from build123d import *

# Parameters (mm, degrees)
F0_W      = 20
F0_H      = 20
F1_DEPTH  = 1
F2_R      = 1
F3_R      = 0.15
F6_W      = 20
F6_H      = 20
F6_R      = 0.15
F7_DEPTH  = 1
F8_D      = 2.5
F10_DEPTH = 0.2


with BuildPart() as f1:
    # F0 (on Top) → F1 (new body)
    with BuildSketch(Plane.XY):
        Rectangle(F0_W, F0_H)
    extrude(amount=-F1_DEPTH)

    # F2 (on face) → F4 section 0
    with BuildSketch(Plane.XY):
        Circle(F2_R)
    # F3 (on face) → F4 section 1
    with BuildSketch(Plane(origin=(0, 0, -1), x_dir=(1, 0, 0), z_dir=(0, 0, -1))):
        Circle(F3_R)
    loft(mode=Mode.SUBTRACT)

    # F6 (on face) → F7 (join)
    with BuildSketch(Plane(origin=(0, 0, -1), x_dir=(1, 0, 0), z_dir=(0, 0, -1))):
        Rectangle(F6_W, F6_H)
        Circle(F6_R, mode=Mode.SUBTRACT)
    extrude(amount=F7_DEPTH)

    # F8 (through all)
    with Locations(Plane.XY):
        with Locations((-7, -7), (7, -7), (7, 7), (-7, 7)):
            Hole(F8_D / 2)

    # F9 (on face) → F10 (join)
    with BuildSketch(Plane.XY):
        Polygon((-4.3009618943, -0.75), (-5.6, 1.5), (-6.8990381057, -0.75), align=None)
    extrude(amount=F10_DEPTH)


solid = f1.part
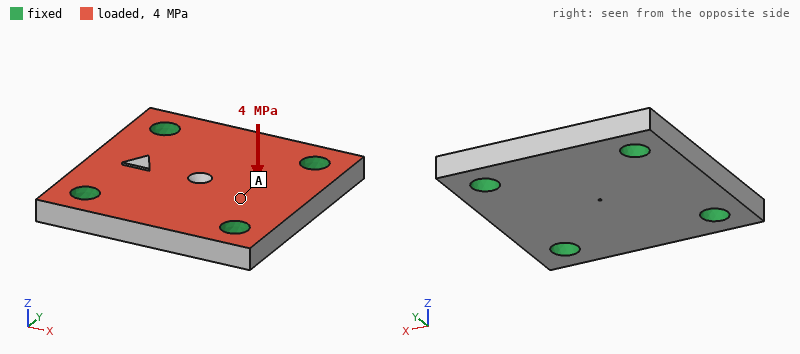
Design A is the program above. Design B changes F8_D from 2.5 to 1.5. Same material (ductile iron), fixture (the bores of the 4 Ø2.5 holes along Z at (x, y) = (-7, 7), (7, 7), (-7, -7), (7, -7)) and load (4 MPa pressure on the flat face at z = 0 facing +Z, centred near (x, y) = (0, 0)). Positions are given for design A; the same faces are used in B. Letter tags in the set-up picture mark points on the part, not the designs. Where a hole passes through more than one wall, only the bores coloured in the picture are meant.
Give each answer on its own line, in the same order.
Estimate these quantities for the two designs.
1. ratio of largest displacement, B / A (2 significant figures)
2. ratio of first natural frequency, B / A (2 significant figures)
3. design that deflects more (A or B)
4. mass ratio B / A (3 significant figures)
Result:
1.4
0.85
B
1.03
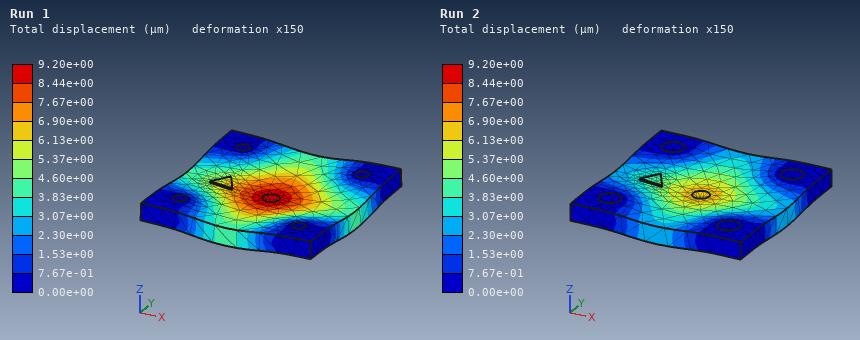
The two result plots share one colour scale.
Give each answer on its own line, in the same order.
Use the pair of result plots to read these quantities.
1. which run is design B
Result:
Run 1
